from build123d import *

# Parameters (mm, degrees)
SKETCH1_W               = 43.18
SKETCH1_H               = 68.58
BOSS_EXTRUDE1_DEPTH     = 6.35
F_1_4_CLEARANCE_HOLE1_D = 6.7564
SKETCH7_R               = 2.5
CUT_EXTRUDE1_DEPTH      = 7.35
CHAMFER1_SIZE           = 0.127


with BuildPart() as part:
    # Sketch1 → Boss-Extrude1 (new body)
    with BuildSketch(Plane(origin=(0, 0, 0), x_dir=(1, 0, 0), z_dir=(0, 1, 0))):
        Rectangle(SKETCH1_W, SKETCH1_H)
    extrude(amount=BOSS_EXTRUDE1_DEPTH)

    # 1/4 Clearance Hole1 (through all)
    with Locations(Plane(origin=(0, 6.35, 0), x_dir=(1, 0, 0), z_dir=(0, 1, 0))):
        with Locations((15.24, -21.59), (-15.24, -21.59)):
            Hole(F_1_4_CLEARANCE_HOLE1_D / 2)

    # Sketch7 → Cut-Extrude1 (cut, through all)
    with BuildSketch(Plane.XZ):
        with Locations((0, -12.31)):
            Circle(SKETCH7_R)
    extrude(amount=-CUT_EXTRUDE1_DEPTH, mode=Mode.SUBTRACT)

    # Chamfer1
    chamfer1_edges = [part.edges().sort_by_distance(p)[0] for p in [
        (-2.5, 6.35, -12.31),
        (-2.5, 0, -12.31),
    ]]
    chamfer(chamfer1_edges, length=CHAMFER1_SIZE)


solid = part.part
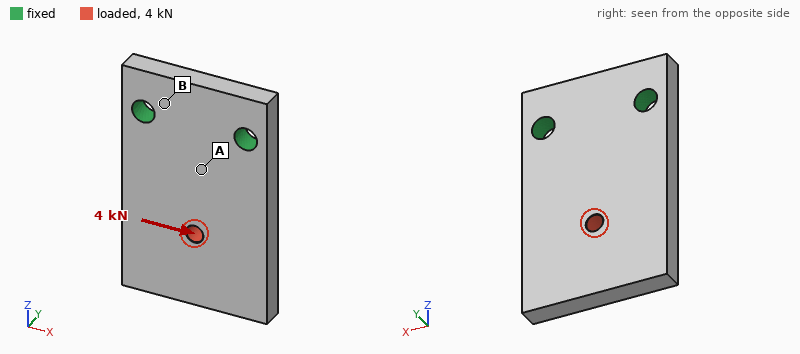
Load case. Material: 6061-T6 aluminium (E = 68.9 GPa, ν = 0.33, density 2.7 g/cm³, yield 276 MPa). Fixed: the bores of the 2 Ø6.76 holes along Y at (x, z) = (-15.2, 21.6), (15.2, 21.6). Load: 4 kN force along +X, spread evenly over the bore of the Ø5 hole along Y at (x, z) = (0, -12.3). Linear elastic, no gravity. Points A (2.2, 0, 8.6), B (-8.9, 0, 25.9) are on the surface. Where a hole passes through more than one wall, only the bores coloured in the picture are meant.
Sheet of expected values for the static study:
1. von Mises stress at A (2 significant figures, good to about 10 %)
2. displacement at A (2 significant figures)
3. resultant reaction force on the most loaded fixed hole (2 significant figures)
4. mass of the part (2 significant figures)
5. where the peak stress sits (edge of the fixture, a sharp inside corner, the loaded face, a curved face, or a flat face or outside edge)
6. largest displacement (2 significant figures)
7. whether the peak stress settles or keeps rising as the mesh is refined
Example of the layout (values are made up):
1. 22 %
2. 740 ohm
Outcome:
1. 35 MPa
2. 10 µm
3. 4.4 kN
4. 49 g
5. edge of the fixture
6. 56 µm
7. keeps rising
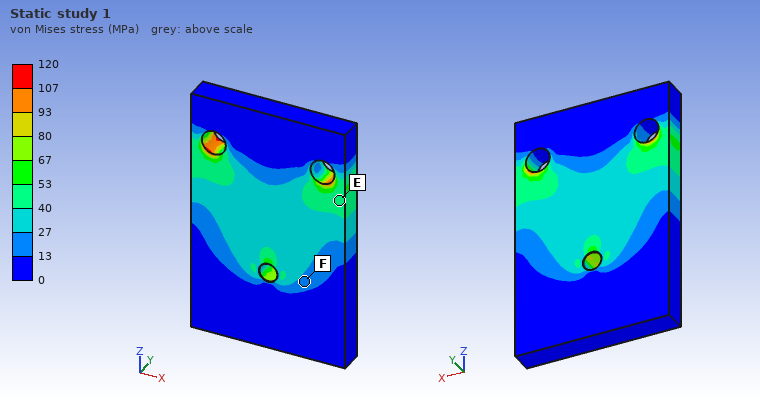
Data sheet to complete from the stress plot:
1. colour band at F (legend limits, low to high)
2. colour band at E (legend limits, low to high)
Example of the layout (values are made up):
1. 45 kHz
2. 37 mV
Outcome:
1. 13 to 27 MPa
2. 40 to 53 MPa
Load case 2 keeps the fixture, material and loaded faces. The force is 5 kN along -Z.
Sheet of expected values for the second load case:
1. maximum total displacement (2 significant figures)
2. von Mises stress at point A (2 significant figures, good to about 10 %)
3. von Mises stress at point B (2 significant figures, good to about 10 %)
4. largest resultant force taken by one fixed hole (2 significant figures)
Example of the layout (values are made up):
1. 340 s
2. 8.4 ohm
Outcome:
1. 15 µm
2. 17 MPa
3. 11 MPa
4. 2.5 kN
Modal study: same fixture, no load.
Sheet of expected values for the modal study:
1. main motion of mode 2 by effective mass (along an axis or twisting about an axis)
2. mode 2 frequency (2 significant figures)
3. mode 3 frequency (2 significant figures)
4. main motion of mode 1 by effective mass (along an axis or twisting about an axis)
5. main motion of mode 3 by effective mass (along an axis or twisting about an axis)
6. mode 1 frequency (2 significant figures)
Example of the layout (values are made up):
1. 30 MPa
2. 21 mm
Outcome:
1. twisting about Z
2. 4900 Hz
3. 8500 Hz
4. along Y
5. along X
6. 1700 Hz
